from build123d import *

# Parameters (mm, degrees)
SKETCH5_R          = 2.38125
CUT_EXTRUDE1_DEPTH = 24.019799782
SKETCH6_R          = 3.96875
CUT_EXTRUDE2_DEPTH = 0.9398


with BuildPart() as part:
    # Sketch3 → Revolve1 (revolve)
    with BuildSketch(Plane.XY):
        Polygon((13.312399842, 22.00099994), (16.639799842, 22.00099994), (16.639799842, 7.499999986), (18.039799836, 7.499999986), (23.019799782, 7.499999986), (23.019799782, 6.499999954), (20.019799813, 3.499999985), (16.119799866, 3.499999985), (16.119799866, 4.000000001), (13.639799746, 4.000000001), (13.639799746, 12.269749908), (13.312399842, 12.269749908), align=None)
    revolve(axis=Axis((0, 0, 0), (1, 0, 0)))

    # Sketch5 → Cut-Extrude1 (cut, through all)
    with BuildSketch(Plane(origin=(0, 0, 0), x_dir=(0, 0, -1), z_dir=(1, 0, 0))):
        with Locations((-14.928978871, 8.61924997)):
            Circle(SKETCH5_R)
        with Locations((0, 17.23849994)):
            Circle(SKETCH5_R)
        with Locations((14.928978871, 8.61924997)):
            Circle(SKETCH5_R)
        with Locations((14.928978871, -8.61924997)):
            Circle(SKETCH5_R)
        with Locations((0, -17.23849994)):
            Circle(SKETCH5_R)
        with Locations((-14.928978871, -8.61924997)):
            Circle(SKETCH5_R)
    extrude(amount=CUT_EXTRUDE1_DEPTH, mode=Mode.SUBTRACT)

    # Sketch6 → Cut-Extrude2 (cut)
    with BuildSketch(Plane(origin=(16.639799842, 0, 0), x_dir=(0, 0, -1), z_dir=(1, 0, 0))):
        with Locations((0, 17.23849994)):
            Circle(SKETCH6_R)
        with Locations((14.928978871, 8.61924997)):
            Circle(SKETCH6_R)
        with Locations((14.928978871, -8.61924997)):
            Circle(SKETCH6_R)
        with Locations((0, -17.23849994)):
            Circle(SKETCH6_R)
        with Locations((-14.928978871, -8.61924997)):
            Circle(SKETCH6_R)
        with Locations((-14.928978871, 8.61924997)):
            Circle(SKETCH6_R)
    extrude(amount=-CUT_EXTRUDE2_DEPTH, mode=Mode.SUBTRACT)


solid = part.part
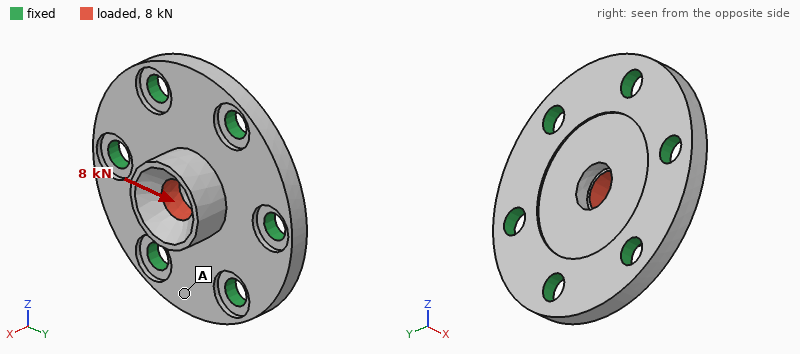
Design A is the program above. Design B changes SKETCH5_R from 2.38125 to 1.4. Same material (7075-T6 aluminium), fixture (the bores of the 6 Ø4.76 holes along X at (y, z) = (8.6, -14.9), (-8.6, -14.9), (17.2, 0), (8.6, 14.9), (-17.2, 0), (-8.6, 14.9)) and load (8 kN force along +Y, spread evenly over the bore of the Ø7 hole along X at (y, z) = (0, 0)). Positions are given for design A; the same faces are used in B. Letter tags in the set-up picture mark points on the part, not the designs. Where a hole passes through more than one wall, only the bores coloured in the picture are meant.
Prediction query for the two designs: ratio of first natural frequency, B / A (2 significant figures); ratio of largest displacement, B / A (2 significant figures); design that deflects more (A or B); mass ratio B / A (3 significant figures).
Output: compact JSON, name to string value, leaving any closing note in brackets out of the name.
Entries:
{"ratio of first natural frequency, B / A": "0.83", "ratio of largest displacement, B / A": "1.2", "design that deflects more": "B", "mass ratio B / A": "1.03"}
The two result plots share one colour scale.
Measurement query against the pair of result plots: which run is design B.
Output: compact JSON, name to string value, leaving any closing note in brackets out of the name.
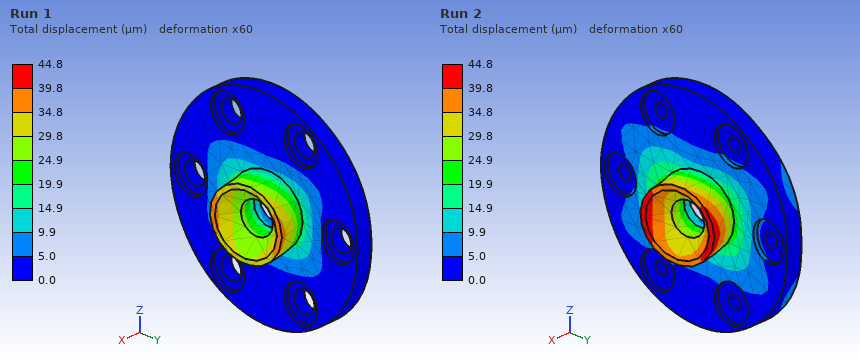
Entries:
{"which run is design B": "Run 2"}
